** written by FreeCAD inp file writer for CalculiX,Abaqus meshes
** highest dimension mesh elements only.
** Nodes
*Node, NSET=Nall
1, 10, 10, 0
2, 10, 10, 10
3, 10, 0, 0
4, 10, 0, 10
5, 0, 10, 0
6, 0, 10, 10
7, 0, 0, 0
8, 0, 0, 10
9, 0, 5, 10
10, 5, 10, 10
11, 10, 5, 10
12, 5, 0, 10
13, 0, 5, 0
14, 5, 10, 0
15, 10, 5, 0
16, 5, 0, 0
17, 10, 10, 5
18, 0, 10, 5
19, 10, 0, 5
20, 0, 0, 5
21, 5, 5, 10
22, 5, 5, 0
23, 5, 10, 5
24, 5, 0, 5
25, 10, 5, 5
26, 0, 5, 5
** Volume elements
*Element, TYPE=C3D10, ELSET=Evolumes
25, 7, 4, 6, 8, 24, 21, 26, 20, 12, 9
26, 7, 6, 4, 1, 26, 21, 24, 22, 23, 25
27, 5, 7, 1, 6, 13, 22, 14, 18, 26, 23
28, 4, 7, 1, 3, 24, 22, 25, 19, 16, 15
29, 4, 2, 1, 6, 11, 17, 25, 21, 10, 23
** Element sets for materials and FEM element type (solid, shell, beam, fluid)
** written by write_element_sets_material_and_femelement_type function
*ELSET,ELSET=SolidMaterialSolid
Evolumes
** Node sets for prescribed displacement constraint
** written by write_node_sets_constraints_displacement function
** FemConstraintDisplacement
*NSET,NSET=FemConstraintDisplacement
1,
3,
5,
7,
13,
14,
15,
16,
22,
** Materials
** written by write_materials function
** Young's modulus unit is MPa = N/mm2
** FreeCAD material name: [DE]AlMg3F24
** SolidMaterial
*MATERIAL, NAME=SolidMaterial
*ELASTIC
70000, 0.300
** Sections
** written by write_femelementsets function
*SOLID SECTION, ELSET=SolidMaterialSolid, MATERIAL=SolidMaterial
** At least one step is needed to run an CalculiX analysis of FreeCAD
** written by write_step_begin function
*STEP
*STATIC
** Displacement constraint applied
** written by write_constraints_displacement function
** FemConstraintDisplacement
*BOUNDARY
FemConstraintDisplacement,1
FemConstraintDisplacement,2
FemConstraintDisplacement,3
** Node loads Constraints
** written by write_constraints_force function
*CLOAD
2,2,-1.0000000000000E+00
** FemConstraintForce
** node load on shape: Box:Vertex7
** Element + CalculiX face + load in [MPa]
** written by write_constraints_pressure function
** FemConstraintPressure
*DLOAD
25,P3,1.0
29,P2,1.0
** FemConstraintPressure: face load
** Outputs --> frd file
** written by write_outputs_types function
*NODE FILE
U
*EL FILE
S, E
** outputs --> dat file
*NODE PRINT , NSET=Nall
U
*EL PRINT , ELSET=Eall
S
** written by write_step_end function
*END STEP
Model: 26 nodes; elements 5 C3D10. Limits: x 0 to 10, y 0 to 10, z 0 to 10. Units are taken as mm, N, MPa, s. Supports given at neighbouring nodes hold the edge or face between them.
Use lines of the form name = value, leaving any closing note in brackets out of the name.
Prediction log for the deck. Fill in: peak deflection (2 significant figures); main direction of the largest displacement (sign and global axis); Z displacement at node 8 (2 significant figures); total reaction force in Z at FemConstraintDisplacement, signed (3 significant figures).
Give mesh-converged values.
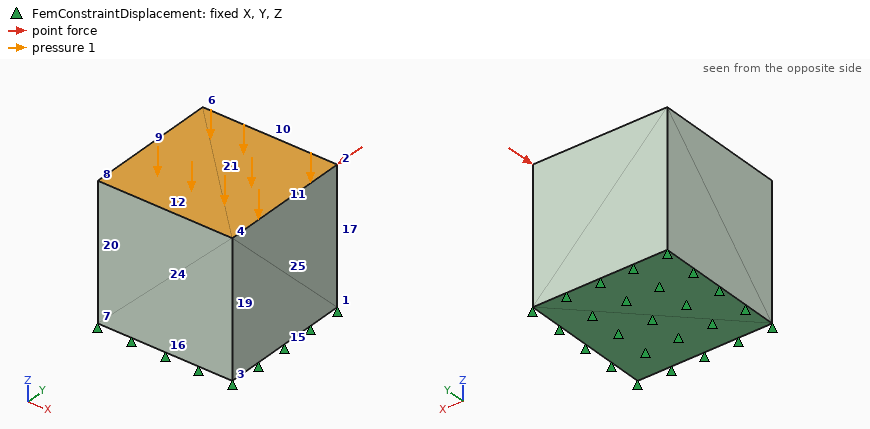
peak deflection = 1.5e-04 mm
main direction of the largest displacement = -Z
Z displacement at node 8 = -1.4e-04 mm
total reaction force in Z at FemConstraintDisplacement, signed = 100 N
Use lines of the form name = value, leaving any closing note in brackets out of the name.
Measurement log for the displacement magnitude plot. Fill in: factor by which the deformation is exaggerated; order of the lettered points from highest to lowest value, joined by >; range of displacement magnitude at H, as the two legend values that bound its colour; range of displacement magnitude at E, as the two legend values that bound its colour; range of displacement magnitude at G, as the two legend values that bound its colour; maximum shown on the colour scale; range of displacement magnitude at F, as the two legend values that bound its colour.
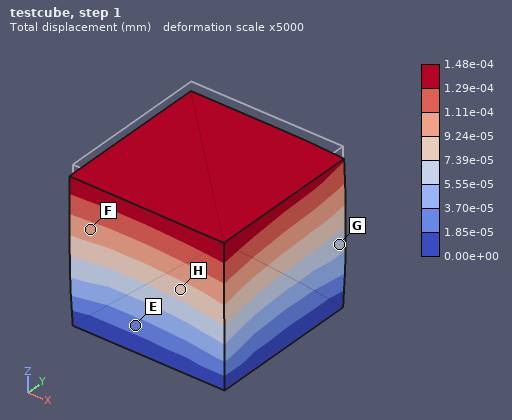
factor by which the deformation is exaggerated = 5000
order of the lettered points from highest to lowest value, joined by > = F > H > G > E
range of displacement magnitude at H, as the two legend values that bound its colour = 7.39e-05 to 9.24e-05 mm
range of displacement magnitude at E, as the two legend values that bound its colour = 1.85e-05 to 3.70e-05 mm
range of displacement magnitude at G, as the two legend values that bound its colour = 5.55e-05 to 7.39e-05 mm
maximum shown on the colour scale = 1.48e-04 mm
range of displacement magnitude at F, as the two legend values that bound its colour = 9.24e-05 to 1.11e-04 mm
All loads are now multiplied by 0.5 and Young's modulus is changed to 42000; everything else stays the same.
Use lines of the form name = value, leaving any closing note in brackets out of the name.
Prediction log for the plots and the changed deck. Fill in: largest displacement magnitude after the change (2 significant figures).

largest displacement magnitude after the change = 1.2e-04 mm
